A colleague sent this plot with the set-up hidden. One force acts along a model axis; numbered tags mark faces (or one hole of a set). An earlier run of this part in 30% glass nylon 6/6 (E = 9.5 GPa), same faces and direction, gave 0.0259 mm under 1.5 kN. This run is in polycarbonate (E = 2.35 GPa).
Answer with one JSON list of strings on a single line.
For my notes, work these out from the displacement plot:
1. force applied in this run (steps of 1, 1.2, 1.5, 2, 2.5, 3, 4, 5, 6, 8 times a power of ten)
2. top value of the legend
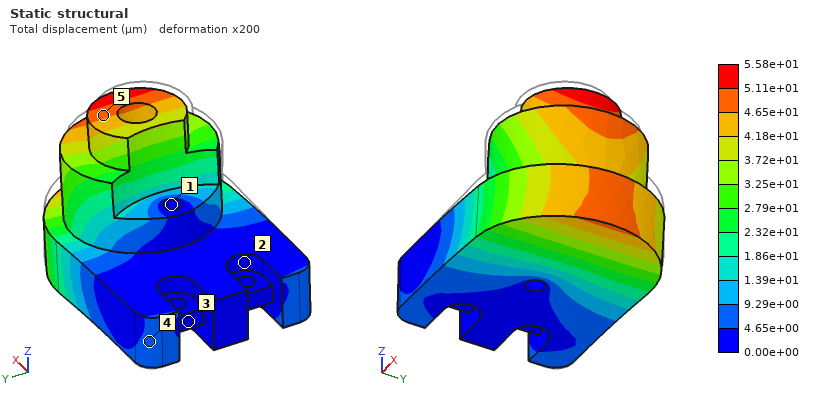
["800 N", "5.58e+01 µm"]
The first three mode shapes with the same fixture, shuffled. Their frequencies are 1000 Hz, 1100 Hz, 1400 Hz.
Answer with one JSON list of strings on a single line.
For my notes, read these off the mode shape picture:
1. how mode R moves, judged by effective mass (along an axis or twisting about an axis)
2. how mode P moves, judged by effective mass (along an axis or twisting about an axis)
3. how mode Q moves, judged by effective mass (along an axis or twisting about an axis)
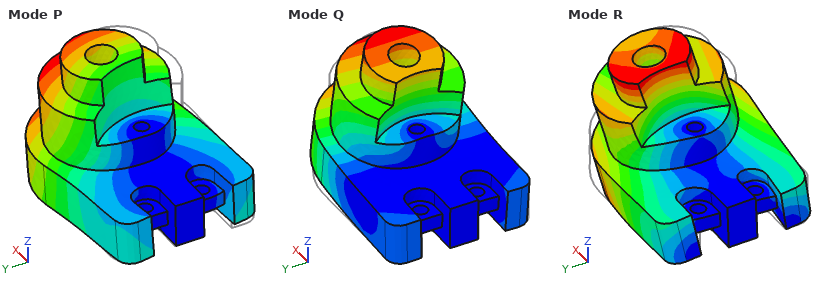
["twisting about X", "along Y", "along Z"]
